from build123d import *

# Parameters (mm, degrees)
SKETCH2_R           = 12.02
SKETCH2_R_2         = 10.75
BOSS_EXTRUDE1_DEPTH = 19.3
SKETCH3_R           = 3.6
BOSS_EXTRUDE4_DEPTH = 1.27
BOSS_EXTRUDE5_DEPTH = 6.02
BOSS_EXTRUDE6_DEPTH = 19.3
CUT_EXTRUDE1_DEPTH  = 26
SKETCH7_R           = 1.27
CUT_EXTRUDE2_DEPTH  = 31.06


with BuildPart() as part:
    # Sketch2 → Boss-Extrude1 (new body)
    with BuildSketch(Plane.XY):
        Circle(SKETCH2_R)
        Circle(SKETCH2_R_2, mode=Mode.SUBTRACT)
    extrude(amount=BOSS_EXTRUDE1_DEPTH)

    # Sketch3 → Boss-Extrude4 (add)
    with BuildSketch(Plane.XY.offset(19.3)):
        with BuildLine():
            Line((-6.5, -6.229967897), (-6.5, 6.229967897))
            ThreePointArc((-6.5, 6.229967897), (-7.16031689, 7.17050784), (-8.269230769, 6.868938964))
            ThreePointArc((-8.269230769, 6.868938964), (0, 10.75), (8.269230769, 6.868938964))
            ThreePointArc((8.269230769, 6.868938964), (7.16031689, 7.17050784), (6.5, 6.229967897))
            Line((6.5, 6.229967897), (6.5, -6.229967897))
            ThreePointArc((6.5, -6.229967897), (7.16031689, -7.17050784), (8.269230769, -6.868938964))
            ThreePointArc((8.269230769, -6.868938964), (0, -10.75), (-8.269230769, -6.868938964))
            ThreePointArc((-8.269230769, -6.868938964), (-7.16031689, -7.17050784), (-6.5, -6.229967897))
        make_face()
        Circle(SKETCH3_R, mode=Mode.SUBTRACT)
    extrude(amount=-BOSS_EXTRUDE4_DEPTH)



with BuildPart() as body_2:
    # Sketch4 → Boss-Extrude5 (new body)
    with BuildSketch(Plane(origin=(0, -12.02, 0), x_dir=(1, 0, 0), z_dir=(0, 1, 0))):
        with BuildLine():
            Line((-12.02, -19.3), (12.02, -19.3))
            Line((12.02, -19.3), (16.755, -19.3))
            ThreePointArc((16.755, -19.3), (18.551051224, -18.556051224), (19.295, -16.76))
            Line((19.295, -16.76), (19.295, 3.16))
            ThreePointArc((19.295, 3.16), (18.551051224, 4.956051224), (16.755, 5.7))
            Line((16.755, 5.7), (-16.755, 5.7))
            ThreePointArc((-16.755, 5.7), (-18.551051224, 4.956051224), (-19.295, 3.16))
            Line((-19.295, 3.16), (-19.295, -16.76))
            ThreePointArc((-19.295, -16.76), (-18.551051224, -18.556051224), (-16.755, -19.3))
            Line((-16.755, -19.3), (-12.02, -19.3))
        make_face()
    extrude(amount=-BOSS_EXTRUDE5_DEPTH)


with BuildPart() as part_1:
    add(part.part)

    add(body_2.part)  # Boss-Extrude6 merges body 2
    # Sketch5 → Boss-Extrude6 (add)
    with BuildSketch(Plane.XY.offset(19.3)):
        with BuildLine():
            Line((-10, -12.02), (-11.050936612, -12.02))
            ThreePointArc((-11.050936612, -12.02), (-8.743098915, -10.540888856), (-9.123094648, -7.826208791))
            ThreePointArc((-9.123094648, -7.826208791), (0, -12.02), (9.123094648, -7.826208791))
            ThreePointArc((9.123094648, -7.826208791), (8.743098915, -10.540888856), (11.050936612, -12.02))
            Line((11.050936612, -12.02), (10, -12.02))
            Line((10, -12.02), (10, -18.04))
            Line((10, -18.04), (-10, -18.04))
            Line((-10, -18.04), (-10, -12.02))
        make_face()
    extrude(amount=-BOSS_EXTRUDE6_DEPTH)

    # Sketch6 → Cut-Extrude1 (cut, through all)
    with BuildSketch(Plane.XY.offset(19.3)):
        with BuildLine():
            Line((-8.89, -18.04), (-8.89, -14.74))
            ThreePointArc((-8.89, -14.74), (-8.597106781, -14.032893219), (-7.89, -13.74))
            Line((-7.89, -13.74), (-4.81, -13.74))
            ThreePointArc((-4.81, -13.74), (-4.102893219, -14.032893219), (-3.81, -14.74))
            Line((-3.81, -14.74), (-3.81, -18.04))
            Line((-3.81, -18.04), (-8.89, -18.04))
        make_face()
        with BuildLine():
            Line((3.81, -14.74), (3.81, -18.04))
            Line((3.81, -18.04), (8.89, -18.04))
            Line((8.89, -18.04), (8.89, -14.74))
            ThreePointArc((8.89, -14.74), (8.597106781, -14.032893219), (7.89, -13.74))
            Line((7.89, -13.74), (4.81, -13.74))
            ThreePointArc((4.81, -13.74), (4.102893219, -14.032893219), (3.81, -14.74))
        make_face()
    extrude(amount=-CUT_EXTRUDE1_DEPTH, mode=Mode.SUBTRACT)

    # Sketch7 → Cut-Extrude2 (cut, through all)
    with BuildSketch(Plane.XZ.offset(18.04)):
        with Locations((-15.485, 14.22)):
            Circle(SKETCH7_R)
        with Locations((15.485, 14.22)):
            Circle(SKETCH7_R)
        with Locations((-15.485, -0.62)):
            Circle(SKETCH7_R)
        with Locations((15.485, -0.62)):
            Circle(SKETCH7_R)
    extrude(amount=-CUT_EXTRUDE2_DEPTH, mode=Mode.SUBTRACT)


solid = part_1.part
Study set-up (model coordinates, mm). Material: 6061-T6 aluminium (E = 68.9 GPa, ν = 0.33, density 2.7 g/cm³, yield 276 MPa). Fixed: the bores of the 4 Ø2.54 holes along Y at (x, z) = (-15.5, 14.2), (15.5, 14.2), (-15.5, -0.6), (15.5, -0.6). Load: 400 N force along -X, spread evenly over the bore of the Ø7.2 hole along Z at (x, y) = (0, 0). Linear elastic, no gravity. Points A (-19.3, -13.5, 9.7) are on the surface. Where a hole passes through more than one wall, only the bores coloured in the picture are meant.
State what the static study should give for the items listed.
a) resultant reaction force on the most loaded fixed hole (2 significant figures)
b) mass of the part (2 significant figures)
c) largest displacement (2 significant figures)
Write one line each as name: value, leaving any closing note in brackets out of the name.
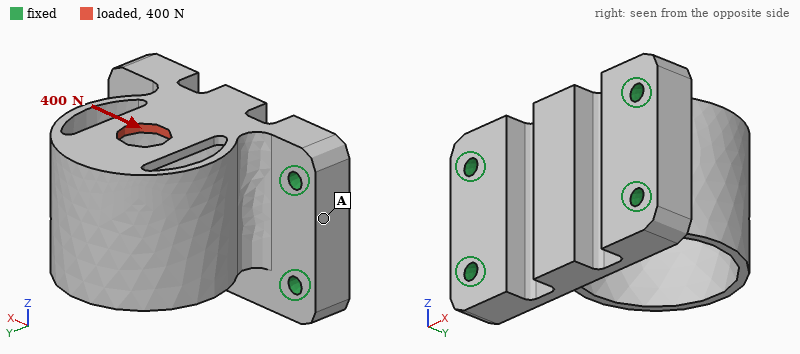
resultant reaction force on the most loaded fixed hole: 300 N
mass of the part: 19 g
largest displacement: 50 µm
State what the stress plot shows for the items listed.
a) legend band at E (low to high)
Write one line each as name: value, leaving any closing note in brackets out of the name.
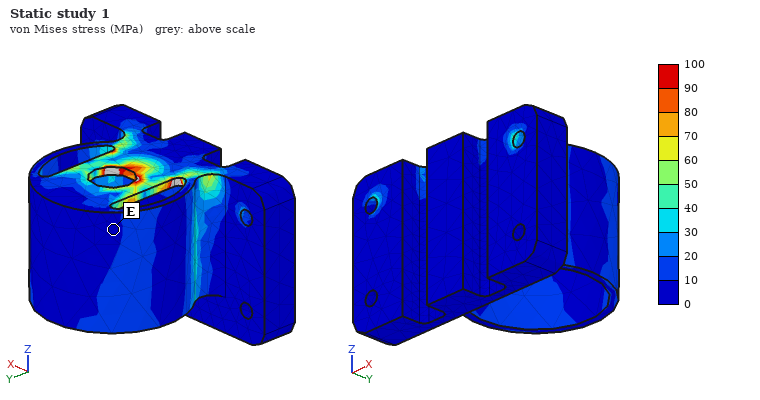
legend band at E: 0 to 10 MPa
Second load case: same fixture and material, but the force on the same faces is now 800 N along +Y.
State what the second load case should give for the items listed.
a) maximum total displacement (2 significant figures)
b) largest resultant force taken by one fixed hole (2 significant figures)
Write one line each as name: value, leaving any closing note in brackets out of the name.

maximum total displacement: 35 µm
largest resultant force taken by one fixed hole: 600 N
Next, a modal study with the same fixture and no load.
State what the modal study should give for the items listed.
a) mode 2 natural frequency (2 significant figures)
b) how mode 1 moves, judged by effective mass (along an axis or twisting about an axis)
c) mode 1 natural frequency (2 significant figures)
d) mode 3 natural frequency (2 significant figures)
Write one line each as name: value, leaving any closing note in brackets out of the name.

mode 2 natural frequency: 6700 Hz
how mode 1 moves, judged by effective mass: along X
mode 1 natural frequency: 5500 Hz
mode 3 natural frequency: 12 kHz
